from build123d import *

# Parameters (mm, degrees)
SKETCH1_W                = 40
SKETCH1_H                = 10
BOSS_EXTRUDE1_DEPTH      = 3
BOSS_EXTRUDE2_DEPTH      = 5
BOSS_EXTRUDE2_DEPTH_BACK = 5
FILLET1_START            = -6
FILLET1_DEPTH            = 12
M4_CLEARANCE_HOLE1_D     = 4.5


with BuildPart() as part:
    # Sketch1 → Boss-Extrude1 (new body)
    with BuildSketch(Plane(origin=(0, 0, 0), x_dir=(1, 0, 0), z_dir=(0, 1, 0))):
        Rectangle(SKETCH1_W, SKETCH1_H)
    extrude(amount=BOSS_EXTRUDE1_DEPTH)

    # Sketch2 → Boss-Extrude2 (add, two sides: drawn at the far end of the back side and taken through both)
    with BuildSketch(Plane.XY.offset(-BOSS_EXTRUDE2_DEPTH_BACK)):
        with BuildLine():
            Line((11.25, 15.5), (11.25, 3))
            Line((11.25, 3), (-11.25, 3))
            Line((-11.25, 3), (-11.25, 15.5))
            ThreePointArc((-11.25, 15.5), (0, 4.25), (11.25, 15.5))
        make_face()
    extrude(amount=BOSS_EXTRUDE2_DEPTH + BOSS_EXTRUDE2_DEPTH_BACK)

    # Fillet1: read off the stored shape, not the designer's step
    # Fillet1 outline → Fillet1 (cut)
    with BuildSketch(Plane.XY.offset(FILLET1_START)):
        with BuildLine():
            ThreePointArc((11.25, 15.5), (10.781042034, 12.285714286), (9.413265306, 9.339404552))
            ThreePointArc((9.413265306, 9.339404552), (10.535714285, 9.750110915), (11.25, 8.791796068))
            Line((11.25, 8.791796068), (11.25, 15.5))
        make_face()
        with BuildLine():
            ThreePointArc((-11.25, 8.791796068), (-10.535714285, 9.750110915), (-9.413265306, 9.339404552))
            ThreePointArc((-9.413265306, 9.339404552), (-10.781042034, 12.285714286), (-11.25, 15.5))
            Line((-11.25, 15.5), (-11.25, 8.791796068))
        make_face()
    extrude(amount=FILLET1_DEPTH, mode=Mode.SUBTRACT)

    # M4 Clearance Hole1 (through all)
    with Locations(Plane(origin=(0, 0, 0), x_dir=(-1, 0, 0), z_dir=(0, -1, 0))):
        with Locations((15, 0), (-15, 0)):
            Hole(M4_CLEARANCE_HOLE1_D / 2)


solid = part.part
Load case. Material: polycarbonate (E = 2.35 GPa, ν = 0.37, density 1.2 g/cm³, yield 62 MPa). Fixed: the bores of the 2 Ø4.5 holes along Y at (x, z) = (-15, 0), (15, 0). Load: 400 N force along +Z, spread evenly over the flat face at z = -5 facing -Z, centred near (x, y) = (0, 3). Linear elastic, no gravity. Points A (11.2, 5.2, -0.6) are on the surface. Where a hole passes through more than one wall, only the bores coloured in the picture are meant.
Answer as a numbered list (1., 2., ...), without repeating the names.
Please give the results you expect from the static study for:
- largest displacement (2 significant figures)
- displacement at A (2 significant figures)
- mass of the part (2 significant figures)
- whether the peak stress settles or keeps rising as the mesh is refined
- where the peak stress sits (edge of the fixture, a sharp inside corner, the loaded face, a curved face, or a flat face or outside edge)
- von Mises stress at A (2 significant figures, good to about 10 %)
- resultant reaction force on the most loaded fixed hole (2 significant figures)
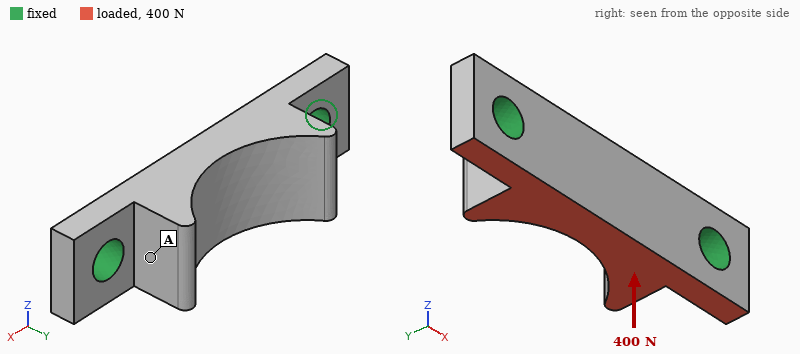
1. 0.13 mm
2. 0.069 mm
3. 2.2 g
4. keeps rising
5. edge of the fixture
6. 4.7 MPa
7. 200 N
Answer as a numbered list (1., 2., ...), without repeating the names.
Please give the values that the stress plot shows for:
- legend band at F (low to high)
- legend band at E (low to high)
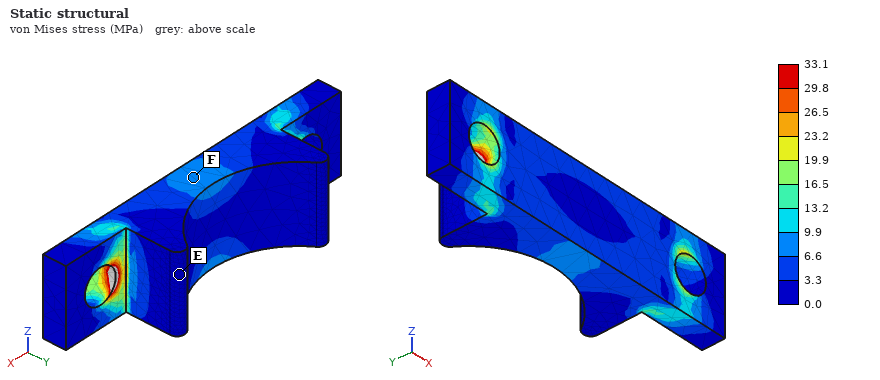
1. 6.6 to 9.9 MPa
2. 0.0 to 3.3 MPa
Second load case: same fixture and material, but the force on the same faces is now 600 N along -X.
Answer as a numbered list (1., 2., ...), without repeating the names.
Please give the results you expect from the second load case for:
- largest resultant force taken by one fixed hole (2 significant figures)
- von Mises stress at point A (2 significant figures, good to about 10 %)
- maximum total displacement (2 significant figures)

1. 310 N
2. 4.8 MPa
3. 85 µm
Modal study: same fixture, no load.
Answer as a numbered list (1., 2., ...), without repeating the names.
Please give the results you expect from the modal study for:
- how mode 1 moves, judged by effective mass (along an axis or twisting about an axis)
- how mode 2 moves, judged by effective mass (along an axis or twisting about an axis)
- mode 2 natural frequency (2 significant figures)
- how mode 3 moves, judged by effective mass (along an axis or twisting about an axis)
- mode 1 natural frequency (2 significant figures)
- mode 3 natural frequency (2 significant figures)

1. along Y
2. along Z
3. 6400 Hz
4. along Z
5. 5400 Hz
6. 9300 Hz
